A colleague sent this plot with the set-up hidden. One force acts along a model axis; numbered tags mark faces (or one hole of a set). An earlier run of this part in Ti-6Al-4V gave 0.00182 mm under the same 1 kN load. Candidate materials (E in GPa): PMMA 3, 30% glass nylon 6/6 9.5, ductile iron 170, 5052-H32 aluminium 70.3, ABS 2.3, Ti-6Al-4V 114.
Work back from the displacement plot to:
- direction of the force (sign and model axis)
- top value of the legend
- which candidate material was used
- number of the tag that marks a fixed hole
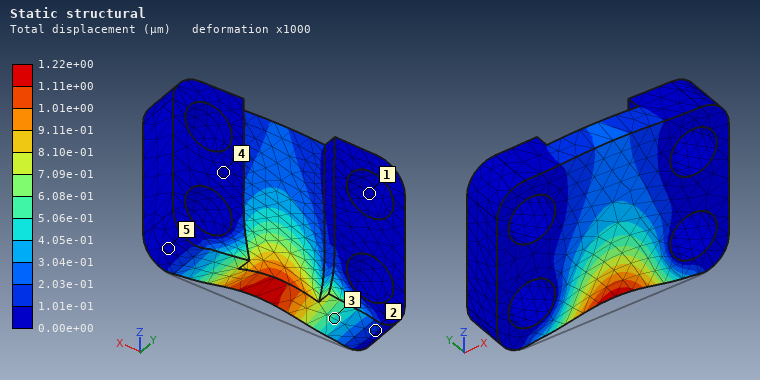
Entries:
+Z
1.22e+00 µm
ductile iron
1
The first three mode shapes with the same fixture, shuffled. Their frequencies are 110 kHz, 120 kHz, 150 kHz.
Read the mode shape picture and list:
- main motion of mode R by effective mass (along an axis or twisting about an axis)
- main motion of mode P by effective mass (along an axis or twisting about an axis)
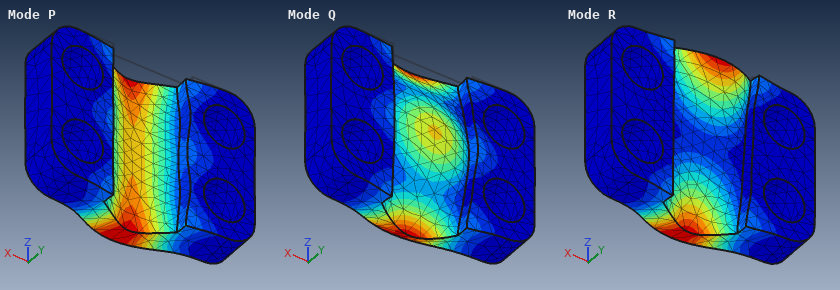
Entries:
twisting about X
along Y
